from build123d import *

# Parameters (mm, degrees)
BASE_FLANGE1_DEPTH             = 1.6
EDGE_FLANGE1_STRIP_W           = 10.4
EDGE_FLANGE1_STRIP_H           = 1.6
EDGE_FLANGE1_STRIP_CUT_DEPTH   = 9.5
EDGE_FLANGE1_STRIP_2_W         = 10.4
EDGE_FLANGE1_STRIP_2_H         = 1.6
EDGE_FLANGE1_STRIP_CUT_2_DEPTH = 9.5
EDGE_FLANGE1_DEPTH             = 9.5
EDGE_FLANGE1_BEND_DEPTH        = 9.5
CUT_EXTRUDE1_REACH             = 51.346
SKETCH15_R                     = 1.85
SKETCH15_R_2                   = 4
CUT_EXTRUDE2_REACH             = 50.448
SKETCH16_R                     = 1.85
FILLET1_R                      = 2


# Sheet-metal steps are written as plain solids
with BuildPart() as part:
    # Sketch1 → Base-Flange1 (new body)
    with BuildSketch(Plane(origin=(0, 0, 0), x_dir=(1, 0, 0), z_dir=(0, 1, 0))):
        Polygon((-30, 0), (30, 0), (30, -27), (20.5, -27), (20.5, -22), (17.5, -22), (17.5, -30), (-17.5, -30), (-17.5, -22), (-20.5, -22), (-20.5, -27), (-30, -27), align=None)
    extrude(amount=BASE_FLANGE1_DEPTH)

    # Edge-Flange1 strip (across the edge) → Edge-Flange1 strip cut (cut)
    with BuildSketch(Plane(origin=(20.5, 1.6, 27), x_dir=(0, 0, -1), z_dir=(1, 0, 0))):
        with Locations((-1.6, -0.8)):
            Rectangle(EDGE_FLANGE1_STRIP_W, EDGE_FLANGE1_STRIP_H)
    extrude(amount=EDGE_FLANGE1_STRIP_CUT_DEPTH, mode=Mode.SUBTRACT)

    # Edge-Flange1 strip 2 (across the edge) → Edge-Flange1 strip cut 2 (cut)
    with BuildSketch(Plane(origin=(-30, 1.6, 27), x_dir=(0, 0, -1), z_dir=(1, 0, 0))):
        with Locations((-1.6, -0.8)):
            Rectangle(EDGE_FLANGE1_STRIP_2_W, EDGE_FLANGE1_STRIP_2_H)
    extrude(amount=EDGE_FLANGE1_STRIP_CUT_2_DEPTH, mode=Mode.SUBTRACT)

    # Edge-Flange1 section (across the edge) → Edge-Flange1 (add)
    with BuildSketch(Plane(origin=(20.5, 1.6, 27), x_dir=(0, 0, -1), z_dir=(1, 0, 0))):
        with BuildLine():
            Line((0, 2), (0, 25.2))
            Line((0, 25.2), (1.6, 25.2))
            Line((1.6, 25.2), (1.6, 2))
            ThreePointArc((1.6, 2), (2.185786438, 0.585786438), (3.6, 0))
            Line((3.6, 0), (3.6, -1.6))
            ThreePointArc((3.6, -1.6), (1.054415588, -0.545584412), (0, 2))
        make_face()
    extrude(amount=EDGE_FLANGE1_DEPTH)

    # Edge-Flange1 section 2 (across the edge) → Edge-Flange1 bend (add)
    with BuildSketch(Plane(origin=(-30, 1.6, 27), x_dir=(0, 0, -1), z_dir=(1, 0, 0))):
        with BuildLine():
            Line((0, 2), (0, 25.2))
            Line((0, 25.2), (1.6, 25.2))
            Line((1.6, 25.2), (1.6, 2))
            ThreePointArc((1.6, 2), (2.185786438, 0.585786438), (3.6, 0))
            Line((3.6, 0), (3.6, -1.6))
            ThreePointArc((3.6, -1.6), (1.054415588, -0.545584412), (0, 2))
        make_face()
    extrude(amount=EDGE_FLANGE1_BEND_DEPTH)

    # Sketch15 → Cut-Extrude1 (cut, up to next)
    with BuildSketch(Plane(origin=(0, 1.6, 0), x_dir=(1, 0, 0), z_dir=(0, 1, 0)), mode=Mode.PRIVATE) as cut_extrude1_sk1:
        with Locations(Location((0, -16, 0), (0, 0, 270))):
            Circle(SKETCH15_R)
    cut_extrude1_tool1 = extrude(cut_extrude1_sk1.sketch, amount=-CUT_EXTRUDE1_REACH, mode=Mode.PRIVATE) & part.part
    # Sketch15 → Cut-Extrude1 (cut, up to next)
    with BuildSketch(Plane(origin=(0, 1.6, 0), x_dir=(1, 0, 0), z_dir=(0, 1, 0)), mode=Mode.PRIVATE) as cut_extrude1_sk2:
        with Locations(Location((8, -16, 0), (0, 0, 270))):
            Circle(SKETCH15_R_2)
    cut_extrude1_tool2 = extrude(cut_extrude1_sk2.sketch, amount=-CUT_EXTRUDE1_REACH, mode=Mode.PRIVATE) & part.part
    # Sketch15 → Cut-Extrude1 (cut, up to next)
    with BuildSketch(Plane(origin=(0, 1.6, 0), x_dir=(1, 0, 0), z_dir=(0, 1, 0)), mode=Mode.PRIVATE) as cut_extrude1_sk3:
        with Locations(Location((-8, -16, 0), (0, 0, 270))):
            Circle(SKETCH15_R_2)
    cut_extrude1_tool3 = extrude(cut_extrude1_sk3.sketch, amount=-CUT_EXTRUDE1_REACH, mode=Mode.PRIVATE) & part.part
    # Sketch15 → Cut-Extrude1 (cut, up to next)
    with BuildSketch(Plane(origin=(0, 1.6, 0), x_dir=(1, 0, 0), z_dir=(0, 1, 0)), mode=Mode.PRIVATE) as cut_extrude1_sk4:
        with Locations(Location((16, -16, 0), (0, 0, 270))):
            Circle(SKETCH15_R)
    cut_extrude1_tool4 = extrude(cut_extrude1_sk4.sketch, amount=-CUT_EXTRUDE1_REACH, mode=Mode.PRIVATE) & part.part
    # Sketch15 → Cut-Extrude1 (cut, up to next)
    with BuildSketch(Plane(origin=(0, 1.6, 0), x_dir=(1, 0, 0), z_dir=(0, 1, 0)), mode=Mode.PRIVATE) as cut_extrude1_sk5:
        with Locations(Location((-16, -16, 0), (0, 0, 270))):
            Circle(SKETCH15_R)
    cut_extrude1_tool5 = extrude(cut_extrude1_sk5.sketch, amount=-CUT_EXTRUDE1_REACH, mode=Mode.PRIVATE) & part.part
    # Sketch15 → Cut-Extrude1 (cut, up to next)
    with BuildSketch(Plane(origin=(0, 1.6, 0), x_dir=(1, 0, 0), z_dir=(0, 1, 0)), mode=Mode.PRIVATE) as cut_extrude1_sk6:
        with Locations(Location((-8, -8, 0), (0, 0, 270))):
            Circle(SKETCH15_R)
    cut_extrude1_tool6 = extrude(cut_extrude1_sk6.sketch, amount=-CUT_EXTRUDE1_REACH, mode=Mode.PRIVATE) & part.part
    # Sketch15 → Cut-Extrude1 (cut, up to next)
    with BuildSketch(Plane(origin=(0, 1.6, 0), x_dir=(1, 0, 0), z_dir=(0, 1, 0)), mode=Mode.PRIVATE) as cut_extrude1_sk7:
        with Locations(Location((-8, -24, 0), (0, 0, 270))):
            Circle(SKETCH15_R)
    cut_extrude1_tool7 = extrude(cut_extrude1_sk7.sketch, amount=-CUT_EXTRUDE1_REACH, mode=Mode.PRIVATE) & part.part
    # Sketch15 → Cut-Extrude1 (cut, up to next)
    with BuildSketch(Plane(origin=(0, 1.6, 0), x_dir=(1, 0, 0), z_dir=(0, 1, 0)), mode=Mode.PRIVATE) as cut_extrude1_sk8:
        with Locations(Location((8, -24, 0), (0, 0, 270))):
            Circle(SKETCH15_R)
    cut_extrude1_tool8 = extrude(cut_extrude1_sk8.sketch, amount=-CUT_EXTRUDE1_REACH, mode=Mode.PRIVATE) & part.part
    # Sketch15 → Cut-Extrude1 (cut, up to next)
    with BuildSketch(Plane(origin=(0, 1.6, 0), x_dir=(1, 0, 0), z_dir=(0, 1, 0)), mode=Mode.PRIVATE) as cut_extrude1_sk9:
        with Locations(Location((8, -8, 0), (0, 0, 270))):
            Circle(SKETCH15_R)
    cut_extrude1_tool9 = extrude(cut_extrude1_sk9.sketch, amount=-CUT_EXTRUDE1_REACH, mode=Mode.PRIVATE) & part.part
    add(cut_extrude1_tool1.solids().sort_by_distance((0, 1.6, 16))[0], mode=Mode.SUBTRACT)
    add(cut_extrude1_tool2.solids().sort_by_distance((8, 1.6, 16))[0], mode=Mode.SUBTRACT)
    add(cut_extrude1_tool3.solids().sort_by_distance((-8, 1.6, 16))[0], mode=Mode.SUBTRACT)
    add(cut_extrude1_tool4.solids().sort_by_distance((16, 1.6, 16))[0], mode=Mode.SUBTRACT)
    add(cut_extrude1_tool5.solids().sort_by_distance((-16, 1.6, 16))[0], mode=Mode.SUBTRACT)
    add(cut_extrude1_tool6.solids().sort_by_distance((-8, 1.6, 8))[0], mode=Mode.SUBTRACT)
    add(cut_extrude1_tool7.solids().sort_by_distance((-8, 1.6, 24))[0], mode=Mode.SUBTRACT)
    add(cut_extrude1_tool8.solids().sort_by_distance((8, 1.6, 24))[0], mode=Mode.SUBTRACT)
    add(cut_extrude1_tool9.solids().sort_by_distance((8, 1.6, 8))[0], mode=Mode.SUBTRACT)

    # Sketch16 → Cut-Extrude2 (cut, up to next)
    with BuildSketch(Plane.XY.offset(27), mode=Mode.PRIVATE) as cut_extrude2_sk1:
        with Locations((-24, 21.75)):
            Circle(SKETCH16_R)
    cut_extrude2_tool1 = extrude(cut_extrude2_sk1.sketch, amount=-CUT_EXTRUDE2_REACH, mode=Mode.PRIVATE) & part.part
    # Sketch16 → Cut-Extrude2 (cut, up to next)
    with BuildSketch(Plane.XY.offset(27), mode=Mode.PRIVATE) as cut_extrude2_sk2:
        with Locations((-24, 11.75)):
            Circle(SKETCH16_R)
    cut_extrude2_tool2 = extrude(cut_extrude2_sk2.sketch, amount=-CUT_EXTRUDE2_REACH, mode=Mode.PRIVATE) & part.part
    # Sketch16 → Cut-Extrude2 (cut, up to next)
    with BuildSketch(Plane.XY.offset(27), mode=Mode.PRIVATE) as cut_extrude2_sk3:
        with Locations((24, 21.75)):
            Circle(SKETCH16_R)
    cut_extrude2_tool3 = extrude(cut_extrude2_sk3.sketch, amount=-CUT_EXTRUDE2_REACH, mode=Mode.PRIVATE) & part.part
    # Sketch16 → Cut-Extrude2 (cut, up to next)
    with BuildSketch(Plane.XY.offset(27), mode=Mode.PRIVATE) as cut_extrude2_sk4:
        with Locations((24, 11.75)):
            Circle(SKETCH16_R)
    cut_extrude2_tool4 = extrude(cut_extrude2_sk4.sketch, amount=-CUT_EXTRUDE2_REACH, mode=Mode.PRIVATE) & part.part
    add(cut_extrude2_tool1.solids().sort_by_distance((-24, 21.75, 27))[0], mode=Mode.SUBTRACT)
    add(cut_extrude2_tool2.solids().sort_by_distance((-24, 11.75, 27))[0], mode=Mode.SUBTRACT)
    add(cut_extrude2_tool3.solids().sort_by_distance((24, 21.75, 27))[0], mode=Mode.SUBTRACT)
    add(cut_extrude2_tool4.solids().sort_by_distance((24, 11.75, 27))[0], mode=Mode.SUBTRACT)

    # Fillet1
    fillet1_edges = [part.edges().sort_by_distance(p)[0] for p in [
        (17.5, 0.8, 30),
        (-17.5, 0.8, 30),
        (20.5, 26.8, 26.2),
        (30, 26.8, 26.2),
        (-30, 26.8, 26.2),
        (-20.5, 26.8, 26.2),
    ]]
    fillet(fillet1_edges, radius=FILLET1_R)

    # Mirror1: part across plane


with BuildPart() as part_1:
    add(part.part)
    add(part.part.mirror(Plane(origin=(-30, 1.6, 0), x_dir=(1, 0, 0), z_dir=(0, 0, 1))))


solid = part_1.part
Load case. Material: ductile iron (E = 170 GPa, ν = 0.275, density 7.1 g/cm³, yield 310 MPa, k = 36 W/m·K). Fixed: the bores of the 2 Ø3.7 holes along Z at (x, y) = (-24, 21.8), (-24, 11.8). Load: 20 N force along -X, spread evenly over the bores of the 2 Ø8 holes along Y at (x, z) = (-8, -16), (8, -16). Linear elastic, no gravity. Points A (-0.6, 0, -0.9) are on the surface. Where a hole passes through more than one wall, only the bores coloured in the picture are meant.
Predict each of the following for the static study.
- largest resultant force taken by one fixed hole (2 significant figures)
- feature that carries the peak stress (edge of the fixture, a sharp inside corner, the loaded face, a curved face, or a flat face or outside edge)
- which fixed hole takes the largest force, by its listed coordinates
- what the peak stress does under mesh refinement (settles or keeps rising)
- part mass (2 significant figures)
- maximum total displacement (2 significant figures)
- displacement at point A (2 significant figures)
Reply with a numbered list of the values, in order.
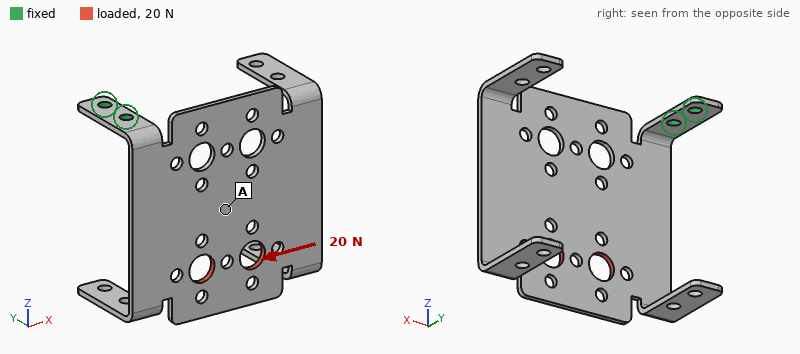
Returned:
1. 30 N
2. edge of the fixture
3. (-24, 11.8)
4. keeps rising
5. 44 g
6. 0.71 mm
7. 0.32 mm
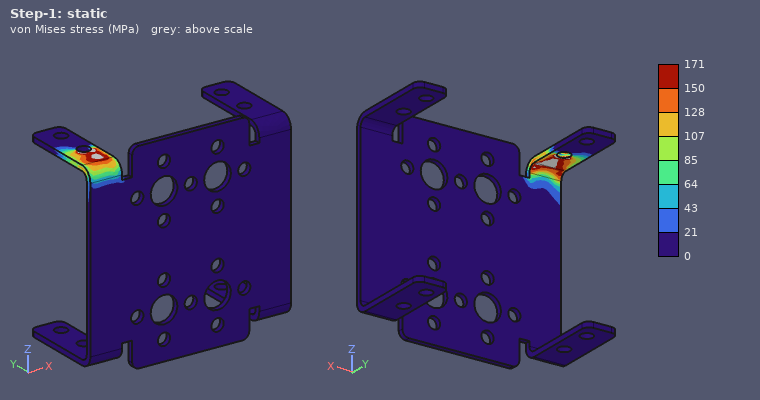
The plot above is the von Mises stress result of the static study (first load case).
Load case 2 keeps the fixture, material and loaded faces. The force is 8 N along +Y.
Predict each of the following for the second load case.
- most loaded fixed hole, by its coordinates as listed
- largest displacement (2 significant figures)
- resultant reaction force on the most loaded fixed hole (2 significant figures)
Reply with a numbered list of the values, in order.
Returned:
1. (-24, 11.8)
2. 0.90 mm
3. 17 N
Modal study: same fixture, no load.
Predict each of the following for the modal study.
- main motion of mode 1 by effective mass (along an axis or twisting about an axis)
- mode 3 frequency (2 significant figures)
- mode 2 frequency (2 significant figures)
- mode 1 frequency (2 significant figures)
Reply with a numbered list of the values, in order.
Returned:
1. along Y
2. 240 Hz
3. 160 Hz
4. 110 Hz
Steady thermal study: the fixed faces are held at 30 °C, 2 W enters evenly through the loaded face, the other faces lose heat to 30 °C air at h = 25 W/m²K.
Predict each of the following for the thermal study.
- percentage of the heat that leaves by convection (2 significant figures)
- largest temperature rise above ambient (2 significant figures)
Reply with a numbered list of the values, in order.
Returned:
1. 93 %
2. 20 K
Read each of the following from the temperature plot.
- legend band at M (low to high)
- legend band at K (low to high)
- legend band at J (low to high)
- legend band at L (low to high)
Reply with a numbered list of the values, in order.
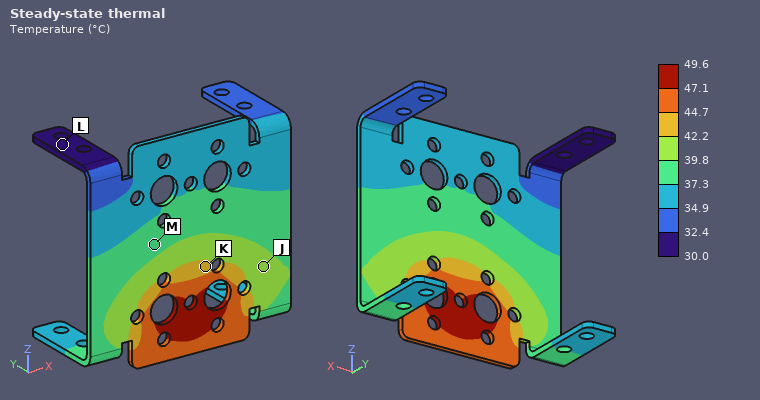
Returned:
1. 37.3 to 39.8 °C
2. 42.2 to 44.7 °C
3. 39.8 to 42.2 °C
4. 30.0 to 32.4 °C
